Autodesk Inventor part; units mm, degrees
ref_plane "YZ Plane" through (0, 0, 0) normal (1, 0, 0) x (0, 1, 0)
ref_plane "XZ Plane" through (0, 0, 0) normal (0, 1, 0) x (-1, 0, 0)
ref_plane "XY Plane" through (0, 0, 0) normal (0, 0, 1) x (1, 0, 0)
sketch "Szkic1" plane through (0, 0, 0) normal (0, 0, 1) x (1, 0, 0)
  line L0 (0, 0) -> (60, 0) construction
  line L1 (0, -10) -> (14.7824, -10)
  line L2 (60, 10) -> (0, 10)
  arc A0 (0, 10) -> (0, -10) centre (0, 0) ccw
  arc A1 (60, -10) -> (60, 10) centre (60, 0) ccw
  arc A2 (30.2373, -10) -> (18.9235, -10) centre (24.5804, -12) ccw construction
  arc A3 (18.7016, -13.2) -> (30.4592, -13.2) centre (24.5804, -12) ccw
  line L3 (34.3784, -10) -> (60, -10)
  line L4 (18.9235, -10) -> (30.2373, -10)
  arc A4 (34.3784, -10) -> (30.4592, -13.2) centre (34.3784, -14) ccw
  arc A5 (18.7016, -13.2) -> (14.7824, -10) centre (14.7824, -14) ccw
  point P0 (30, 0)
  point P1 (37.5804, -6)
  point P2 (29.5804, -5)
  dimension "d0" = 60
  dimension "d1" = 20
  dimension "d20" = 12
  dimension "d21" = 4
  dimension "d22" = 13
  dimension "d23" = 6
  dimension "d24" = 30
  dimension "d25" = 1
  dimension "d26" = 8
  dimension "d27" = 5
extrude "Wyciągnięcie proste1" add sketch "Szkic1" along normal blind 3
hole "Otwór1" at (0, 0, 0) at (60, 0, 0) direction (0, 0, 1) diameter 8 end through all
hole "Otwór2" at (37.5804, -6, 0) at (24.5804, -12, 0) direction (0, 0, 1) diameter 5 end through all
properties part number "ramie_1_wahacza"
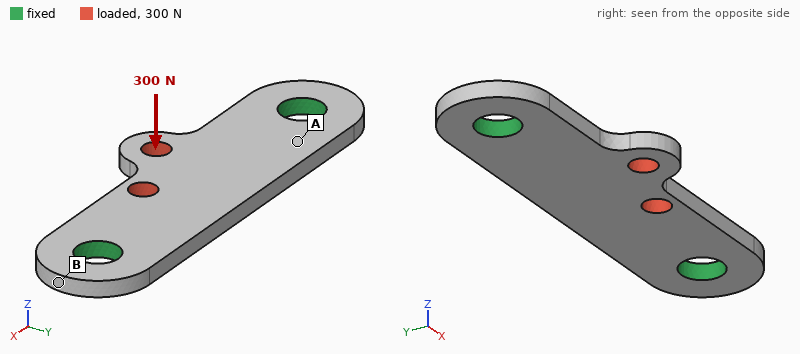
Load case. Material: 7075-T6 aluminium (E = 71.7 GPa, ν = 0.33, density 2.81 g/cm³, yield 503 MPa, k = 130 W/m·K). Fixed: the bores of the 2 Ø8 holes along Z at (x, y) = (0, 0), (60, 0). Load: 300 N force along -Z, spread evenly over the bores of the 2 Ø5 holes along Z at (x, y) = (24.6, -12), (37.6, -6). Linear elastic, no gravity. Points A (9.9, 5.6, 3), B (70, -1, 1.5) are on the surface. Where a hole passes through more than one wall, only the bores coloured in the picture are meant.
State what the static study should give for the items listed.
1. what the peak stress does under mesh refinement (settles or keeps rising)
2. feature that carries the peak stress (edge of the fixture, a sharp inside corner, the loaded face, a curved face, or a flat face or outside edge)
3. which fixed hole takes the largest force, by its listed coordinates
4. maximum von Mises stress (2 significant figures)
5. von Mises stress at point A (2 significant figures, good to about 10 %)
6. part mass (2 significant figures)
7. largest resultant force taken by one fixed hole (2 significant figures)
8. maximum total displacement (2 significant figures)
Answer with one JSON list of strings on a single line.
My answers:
["settles", "the loaded face", "(60, 0)", "160 MPa", "38 MPa", "12 g", "160 N", "0.19 mm"]
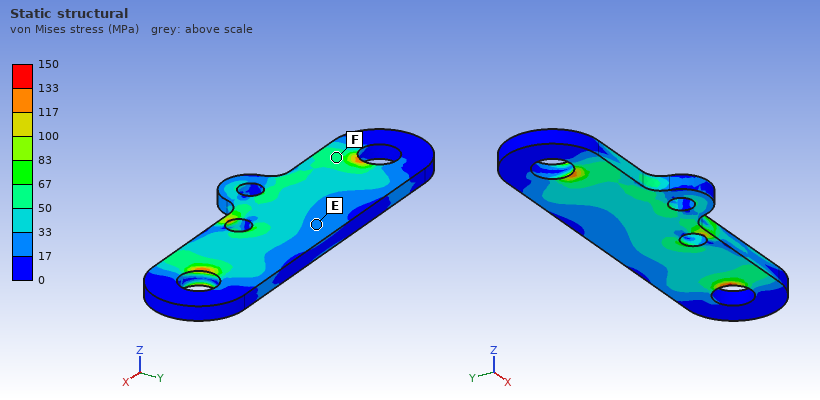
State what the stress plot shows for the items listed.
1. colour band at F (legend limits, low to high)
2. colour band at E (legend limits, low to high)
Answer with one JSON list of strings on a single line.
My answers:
["50 to 67 MPa", "17 to 33 MPa"]
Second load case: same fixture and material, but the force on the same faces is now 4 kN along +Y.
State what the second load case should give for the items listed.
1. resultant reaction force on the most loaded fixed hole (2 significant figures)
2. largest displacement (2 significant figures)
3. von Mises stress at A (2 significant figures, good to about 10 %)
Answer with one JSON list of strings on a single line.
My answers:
["2.1 kN", "73 µm", "56 MPa"]
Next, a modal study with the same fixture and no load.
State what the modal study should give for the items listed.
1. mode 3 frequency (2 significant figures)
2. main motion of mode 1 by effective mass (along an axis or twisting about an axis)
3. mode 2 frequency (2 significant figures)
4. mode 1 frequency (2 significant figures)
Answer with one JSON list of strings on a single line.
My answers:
["13 kHz", "along Z", "7100 Hz", "4800 Hz"]
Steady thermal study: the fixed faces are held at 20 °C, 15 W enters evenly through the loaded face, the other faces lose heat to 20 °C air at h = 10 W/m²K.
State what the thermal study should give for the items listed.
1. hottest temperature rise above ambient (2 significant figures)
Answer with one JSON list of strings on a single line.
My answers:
["34 K"]
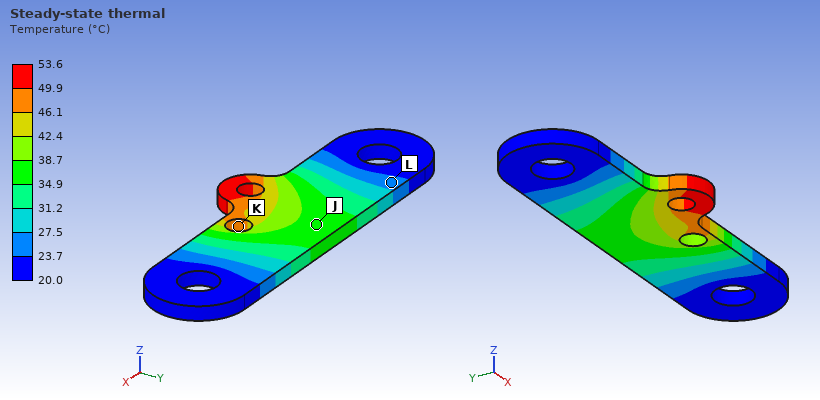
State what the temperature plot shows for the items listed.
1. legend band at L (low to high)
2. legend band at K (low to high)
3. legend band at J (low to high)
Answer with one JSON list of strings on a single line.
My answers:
["23.7 to 27.5 °C", "46.1 to 49.9 °C", "34.9 to 38.7 °C"]
